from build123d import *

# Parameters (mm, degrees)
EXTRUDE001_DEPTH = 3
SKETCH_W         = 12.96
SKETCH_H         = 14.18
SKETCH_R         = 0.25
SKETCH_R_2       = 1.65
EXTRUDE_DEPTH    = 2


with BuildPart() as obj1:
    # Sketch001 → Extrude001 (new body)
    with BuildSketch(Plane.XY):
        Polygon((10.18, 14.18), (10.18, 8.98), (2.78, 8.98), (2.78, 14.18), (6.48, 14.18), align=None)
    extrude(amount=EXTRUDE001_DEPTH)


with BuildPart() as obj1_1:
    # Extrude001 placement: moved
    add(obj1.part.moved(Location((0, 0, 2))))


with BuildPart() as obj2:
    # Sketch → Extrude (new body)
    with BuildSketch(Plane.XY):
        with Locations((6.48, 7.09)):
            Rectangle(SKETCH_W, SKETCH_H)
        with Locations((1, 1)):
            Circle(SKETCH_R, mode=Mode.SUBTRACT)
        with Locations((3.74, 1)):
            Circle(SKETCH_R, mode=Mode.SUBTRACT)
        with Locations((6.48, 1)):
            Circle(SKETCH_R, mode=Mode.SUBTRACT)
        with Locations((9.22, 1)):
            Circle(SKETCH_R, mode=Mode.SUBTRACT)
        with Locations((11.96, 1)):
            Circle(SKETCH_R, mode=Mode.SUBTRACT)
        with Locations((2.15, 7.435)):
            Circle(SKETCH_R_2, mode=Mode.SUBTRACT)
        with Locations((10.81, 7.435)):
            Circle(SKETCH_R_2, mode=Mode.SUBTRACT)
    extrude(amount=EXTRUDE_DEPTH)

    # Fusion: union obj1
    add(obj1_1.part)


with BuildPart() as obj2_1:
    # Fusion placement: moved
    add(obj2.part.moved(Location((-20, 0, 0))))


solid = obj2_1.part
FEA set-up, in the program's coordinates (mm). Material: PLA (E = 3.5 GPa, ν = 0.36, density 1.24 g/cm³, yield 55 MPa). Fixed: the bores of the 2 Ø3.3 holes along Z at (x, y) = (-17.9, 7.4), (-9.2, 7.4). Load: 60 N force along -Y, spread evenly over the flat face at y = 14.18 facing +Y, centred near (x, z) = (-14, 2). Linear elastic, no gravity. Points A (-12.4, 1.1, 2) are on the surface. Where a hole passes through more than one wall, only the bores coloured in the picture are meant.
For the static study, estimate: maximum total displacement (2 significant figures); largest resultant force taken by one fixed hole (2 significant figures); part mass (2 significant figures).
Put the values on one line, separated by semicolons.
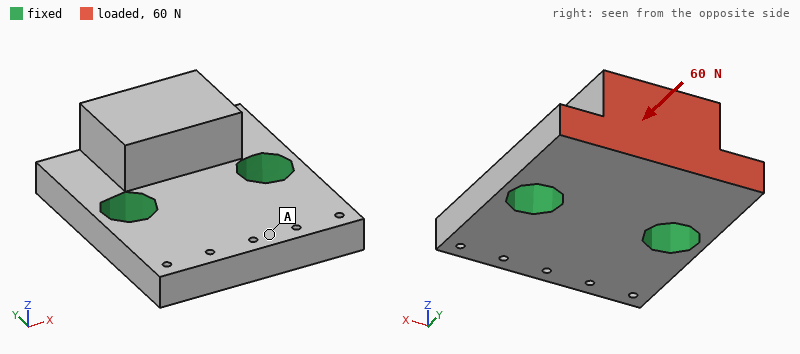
27 µm; 31 N; 0.55 g
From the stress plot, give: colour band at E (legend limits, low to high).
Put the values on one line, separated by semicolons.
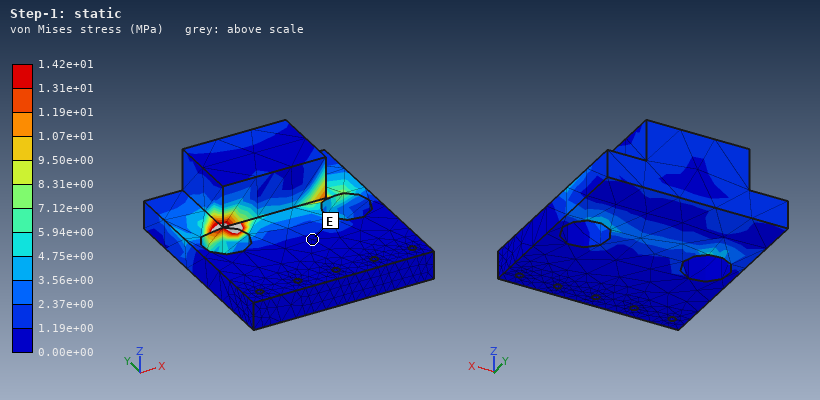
0.00e+00 to 1.19e+00 MPa
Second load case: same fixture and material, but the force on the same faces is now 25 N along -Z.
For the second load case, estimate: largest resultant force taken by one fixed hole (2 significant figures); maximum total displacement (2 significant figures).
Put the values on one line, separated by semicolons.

13 N; 49 µm
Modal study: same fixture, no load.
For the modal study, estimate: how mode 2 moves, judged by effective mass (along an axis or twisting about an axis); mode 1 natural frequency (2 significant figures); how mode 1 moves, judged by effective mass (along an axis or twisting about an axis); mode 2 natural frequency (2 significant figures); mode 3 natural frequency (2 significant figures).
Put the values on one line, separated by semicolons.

along Z; 11 kHz; along Z; 13 kHz; 19 kHz
